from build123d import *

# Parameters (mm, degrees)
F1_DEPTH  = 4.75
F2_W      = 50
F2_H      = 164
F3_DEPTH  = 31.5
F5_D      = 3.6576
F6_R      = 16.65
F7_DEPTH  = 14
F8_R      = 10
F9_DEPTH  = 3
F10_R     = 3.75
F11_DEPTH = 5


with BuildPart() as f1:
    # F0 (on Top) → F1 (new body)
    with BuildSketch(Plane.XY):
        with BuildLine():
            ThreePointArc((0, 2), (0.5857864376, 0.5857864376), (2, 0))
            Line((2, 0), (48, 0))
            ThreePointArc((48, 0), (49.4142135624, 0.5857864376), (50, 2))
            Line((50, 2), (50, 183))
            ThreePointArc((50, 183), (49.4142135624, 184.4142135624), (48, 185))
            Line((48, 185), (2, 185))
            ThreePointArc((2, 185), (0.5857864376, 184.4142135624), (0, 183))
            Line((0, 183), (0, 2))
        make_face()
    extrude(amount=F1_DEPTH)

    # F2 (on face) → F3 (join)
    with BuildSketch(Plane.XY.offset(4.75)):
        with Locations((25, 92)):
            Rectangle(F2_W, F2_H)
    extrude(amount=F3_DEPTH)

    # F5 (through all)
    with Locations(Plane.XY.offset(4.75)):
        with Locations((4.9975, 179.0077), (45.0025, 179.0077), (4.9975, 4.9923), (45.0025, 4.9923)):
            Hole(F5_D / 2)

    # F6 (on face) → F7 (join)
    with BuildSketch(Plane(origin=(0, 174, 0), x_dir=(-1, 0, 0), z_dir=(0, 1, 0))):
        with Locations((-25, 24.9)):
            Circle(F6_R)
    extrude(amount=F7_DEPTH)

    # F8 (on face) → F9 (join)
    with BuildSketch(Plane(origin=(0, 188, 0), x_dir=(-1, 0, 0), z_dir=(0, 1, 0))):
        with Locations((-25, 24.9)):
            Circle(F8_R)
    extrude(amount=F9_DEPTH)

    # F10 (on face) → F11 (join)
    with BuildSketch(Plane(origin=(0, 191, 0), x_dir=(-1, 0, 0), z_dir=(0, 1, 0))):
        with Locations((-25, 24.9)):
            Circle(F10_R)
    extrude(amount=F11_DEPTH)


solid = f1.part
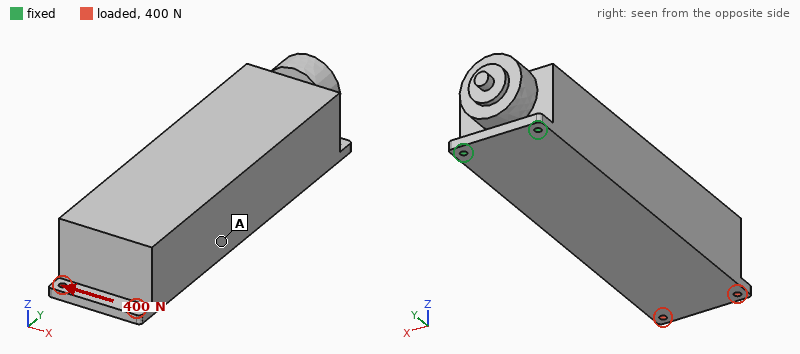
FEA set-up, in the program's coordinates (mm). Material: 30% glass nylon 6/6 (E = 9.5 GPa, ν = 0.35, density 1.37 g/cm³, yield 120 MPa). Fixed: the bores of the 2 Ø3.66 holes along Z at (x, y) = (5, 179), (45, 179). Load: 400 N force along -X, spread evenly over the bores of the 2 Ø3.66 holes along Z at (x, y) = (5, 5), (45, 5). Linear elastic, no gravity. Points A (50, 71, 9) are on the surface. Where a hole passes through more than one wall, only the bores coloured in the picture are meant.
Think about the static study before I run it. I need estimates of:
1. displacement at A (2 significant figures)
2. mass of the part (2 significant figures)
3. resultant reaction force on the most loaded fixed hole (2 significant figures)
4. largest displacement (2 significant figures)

0.35 mm
430 g
1.7 kN
0.65 mm
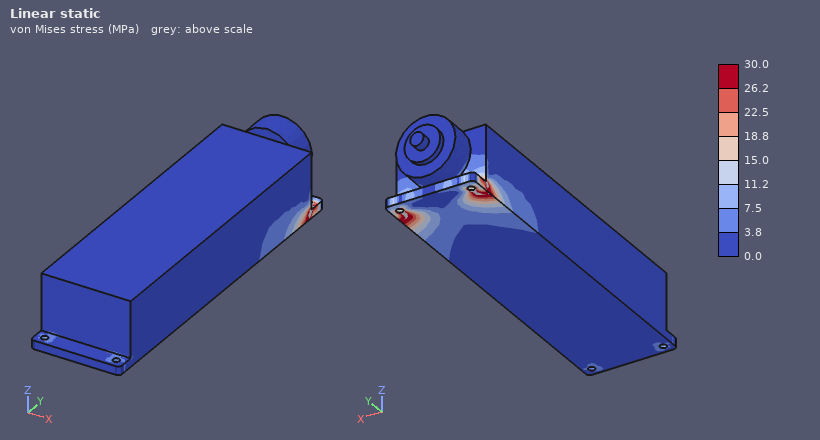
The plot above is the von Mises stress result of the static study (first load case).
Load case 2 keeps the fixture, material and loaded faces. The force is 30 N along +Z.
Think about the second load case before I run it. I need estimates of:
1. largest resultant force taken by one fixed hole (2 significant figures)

16 N
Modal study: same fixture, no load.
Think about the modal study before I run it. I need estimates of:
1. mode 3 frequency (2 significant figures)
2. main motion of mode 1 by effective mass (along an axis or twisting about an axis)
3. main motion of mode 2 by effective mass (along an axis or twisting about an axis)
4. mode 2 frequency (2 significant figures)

1100 Hz
along Z
along X
380 Hz
